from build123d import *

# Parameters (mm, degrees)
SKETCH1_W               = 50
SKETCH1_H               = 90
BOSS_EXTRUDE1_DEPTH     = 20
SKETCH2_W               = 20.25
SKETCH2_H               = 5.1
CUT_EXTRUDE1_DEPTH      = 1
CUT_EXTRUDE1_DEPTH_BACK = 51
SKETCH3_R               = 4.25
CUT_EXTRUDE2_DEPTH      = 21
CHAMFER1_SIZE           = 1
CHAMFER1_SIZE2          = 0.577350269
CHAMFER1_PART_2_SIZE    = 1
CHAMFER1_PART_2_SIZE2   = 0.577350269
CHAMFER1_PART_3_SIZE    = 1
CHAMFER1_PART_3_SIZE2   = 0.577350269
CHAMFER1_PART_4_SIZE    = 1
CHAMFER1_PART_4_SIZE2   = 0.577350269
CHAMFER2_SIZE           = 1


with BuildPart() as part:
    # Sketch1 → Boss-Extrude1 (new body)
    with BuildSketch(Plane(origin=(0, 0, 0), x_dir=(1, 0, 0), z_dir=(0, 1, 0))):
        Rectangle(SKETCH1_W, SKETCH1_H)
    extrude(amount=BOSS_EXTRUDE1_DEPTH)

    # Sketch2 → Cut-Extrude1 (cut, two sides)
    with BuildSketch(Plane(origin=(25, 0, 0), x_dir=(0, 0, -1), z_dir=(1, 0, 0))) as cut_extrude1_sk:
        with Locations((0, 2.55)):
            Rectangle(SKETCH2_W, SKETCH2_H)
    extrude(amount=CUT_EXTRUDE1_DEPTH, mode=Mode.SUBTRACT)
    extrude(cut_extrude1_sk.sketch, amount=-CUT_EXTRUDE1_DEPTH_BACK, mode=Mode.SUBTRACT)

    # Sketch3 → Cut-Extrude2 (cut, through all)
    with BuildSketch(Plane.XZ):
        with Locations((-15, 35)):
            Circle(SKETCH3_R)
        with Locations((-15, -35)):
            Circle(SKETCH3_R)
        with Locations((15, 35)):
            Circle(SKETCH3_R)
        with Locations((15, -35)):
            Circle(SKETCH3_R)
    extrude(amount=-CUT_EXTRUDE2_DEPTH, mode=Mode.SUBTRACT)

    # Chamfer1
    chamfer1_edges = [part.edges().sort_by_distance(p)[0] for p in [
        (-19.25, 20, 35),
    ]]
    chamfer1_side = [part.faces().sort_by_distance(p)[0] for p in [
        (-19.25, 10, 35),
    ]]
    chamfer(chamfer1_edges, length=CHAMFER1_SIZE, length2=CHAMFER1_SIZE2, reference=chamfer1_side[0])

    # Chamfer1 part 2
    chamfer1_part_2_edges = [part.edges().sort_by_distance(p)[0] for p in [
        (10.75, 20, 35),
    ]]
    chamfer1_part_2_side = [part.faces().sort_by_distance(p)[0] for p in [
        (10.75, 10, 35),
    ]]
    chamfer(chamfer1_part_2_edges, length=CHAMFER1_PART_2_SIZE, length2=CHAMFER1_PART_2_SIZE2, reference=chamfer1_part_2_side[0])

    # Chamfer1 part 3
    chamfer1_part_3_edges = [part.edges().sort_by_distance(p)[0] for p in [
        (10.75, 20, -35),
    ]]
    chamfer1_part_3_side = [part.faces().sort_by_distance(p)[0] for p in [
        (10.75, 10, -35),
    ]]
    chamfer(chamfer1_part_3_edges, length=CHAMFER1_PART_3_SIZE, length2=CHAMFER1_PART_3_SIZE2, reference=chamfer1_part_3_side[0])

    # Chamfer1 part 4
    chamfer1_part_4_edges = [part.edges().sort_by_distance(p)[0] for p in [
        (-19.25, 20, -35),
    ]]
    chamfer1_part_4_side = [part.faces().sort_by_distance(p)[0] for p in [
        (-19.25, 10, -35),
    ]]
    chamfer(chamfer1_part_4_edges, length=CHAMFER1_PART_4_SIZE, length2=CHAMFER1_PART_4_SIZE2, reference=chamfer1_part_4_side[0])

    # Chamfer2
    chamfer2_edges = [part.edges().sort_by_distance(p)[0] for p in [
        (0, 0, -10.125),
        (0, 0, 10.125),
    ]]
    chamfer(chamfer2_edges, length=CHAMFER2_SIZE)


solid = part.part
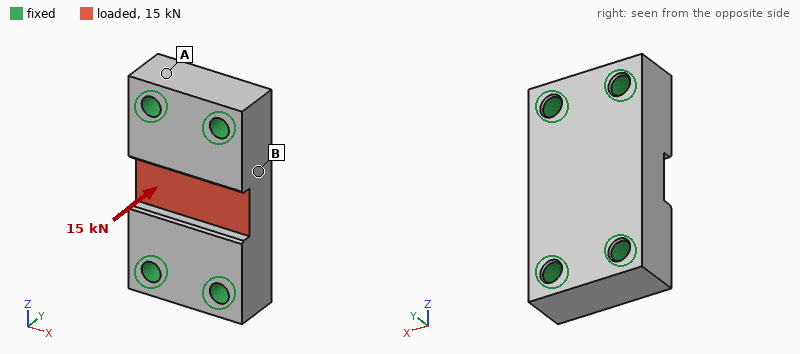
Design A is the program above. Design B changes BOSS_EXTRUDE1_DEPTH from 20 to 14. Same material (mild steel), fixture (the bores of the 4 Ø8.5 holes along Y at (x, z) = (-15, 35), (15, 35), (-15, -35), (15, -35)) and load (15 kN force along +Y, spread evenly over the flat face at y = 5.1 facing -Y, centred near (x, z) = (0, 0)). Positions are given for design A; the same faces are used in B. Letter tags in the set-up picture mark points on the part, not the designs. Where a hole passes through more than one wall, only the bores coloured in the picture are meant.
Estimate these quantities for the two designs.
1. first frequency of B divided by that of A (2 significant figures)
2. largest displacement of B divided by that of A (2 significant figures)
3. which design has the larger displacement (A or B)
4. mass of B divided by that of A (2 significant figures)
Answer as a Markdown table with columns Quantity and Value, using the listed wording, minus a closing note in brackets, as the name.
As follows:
| Quantity | Value |
|---|---|
| first frequency of B divided by that of A | 0.83 |
| largest displacement of B divided by that of A | 2.4 |
| which design has the larger displacement | B |
| mass of B divided by that of A | 0.68 |
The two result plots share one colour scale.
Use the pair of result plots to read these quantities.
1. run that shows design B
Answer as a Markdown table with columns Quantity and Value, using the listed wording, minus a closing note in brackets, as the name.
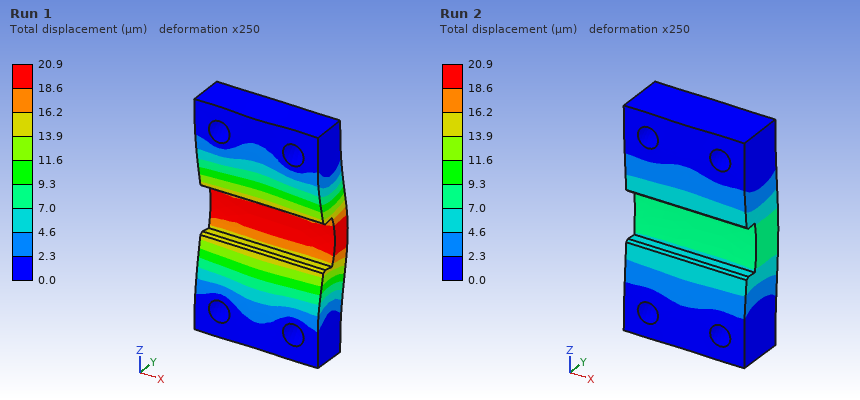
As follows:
| Quantity | Value |
|---|---|
| run that shows design B | Run 1 |
